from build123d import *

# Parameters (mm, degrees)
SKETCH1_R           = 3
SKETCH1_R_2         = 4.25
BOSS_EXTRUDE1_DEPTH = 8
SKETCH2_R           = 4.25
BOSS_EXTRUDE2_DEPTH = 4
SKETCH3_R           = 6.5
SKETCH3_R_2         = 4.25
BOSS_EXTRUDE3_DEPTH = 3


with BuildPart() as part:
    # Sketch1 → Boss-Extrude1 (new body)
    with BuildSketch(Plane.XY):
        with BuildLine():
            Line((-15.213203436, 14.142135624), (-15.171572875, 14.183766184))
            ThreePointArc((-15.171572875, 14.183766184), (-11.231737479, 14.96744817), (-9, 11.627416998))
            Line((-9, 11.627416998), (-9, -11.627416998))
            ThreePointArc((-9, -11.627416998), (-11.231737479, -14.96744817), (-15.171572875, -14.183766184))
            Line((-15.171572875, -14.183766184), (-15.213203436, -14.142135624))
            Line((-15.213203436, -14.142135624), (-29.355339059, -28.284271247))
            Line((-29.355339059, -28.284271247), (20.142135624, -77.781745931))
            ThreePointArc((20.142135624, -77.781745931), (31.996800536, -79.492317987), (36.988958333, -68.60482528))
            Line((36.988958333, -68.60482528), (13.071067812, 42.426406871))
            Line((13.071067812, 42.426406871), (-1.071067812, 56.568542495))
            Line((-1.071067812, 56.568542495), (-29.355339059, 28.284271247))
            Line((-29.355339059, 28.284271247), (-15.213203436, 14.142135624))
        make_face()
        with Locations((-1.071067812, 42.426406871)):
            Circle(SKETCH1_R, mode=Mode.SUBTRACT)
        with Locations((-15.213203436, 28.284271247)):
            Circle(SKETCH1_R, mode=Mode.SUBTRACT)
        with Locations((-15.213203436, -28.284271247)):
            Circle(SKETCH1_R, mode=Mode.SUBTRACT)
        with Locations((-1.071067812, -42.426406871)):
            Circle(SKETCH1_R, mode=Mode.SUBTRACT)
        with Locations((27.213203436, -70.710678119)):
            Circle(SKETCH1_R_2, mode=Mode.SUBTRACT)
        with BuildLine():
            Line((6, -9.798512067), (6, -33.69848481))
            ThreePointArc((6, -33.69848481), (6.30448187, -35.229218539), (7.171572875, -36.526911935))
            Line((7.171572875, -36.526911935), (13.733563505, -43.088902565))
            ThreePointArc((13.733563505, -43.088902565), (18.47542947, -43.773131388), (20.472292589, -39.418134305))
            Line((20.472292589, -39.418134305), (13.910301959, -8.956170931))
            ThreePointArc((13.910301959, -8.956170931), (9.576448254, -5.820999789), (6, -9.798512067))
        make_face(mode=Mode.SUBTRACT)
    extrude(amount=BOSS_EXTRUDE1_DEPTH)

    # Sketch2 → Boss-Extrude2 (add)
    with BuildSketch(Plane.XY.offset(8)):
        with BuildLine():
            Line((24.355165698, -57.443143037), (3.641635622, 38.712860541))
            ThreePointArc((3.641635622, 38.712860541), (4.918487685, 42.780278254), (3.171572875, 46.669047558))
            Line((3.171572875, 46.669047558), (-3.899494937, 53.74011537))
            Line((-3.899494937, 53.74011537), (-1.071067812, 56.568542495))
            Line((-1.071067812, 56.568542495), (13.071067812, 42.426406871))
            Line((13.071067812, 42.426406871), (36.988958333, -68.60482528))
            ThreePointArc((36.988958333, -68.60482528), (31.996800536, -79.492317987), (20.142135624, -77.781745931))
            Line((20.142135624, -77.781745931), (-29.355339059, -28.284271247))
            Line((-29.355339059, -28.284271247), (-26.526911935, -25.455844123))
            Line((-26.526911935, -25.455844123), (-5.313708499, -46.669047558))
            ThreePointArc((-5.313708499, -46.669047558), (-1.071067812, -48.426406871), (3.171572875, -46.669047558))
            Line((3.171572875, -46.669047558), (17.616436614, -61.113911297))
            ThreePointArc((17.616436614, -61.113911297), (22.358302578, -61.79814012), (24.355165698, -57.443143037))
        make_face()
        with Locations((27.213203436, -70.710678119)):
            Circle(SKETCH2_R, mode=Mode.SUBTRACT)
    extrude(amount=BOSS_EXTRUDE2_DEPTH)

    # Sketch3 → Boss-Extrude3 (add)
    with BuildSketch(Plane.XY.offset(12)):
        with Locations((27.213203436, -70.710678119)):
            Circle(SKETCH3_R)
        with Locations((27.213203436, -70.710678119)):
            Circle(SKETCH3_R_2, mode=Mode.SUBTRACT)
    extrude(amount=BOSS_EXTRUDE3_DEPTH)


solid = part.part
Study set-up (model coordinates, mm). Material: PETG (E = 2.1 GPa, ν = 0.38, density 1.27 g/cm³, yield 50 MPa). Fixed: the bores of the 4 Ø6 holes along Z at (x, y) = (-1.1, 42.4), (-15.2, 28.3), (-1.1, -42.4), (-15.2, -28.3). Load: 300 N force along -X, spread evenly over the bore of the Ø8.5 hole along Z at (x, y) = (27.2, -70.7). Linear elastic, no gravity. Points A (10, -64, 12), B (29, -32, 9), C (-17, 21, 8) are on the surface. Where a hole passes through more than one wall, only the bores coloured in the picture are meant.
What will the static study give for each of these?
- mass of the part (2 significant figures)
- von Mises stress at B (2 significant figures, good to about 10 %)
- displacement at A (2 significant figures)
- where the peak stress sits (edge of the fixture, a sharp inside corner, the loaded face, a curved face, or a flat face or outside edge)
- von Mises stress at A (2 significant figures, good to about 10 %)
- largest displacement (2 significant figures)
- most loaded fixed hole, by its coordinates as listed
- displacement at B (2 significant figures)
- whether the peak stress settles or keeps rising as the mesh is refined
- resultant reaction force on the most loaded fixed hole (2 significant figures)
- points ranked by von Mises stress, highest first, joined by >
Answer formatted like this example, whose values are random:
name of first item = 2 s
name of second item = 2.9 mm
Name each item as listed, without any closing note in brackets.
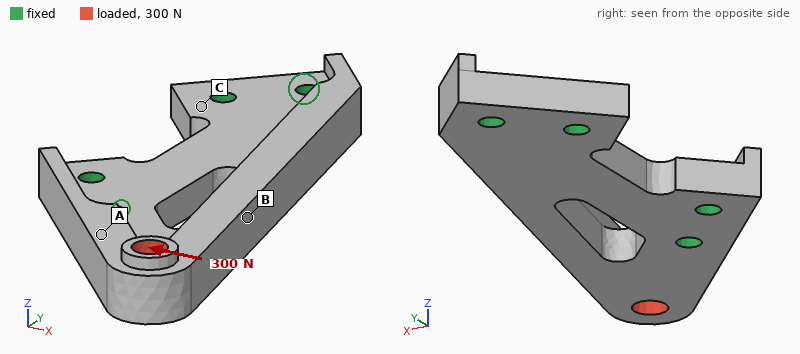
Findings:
mass of the part = 52 g
von Mises stress at B = 2.5 MPa
displacement at A = 0.12 mm
where the peak stress sits = edge of the fixture
von Mises stress at A = 3.8 MPa
largest displacement = 0.29 mm
most loaded fixed hole, by its coordinates as listed = (-1.1, -42.4)
displacement at B = 0.088 mm
whether the peak stress settles or keeps rising as the mesh is refined = keeps rising
resultant reaction force on the most loaded fixed hole = 370 N
points ranked by von Mises stress, highest first, joined by > = A > B > C
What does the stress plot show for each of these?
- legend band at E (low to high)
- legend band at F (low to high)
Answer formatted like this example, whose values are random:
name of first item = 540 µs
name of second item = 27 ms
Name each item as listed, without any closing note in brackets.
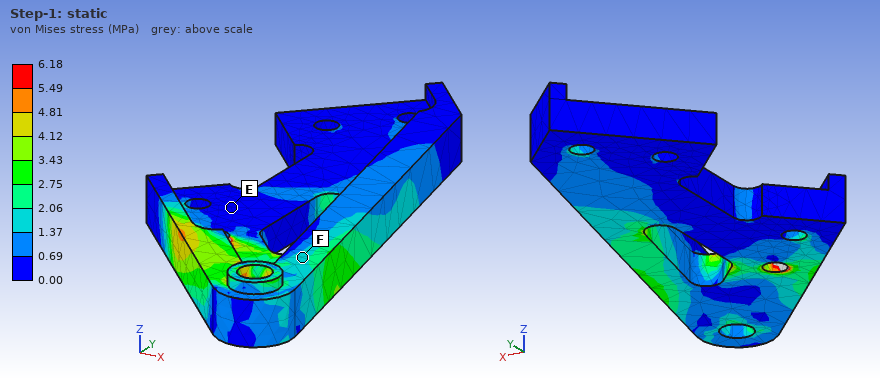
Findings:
legend band at E = 0.00 to 0.69 MPa
legend band at F = 1.37 to 2.06 MPa
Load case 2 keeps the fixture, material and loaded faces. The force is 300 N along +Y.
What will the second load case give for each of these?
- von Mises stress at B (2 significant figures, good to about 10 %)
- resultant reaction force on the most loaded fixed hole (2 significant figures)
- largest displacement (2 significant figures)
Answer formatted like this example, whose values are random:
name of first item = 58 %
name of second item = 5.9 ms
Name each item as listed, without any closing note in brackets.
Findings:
von Mises stress at B = 3.2 MPa
resultant reaction force on the most loaded fixed hole = 150 N
largest displacement = 0.20 mm
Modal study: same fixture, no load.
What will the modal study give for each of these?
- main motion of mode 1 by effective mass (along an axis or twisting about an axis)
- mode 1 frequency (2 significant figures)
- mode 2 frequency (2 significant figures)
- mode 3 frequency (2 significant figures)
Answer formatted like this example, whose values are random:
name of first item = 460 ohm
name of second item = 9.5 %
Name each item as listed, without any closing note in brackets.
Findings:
main motion of mode 1 by effective mass = along Z
mode 1 frequency = 800 Hz
mode 2 frequency = 1200 Hz
mode 3 frequency = 2100 Hz
